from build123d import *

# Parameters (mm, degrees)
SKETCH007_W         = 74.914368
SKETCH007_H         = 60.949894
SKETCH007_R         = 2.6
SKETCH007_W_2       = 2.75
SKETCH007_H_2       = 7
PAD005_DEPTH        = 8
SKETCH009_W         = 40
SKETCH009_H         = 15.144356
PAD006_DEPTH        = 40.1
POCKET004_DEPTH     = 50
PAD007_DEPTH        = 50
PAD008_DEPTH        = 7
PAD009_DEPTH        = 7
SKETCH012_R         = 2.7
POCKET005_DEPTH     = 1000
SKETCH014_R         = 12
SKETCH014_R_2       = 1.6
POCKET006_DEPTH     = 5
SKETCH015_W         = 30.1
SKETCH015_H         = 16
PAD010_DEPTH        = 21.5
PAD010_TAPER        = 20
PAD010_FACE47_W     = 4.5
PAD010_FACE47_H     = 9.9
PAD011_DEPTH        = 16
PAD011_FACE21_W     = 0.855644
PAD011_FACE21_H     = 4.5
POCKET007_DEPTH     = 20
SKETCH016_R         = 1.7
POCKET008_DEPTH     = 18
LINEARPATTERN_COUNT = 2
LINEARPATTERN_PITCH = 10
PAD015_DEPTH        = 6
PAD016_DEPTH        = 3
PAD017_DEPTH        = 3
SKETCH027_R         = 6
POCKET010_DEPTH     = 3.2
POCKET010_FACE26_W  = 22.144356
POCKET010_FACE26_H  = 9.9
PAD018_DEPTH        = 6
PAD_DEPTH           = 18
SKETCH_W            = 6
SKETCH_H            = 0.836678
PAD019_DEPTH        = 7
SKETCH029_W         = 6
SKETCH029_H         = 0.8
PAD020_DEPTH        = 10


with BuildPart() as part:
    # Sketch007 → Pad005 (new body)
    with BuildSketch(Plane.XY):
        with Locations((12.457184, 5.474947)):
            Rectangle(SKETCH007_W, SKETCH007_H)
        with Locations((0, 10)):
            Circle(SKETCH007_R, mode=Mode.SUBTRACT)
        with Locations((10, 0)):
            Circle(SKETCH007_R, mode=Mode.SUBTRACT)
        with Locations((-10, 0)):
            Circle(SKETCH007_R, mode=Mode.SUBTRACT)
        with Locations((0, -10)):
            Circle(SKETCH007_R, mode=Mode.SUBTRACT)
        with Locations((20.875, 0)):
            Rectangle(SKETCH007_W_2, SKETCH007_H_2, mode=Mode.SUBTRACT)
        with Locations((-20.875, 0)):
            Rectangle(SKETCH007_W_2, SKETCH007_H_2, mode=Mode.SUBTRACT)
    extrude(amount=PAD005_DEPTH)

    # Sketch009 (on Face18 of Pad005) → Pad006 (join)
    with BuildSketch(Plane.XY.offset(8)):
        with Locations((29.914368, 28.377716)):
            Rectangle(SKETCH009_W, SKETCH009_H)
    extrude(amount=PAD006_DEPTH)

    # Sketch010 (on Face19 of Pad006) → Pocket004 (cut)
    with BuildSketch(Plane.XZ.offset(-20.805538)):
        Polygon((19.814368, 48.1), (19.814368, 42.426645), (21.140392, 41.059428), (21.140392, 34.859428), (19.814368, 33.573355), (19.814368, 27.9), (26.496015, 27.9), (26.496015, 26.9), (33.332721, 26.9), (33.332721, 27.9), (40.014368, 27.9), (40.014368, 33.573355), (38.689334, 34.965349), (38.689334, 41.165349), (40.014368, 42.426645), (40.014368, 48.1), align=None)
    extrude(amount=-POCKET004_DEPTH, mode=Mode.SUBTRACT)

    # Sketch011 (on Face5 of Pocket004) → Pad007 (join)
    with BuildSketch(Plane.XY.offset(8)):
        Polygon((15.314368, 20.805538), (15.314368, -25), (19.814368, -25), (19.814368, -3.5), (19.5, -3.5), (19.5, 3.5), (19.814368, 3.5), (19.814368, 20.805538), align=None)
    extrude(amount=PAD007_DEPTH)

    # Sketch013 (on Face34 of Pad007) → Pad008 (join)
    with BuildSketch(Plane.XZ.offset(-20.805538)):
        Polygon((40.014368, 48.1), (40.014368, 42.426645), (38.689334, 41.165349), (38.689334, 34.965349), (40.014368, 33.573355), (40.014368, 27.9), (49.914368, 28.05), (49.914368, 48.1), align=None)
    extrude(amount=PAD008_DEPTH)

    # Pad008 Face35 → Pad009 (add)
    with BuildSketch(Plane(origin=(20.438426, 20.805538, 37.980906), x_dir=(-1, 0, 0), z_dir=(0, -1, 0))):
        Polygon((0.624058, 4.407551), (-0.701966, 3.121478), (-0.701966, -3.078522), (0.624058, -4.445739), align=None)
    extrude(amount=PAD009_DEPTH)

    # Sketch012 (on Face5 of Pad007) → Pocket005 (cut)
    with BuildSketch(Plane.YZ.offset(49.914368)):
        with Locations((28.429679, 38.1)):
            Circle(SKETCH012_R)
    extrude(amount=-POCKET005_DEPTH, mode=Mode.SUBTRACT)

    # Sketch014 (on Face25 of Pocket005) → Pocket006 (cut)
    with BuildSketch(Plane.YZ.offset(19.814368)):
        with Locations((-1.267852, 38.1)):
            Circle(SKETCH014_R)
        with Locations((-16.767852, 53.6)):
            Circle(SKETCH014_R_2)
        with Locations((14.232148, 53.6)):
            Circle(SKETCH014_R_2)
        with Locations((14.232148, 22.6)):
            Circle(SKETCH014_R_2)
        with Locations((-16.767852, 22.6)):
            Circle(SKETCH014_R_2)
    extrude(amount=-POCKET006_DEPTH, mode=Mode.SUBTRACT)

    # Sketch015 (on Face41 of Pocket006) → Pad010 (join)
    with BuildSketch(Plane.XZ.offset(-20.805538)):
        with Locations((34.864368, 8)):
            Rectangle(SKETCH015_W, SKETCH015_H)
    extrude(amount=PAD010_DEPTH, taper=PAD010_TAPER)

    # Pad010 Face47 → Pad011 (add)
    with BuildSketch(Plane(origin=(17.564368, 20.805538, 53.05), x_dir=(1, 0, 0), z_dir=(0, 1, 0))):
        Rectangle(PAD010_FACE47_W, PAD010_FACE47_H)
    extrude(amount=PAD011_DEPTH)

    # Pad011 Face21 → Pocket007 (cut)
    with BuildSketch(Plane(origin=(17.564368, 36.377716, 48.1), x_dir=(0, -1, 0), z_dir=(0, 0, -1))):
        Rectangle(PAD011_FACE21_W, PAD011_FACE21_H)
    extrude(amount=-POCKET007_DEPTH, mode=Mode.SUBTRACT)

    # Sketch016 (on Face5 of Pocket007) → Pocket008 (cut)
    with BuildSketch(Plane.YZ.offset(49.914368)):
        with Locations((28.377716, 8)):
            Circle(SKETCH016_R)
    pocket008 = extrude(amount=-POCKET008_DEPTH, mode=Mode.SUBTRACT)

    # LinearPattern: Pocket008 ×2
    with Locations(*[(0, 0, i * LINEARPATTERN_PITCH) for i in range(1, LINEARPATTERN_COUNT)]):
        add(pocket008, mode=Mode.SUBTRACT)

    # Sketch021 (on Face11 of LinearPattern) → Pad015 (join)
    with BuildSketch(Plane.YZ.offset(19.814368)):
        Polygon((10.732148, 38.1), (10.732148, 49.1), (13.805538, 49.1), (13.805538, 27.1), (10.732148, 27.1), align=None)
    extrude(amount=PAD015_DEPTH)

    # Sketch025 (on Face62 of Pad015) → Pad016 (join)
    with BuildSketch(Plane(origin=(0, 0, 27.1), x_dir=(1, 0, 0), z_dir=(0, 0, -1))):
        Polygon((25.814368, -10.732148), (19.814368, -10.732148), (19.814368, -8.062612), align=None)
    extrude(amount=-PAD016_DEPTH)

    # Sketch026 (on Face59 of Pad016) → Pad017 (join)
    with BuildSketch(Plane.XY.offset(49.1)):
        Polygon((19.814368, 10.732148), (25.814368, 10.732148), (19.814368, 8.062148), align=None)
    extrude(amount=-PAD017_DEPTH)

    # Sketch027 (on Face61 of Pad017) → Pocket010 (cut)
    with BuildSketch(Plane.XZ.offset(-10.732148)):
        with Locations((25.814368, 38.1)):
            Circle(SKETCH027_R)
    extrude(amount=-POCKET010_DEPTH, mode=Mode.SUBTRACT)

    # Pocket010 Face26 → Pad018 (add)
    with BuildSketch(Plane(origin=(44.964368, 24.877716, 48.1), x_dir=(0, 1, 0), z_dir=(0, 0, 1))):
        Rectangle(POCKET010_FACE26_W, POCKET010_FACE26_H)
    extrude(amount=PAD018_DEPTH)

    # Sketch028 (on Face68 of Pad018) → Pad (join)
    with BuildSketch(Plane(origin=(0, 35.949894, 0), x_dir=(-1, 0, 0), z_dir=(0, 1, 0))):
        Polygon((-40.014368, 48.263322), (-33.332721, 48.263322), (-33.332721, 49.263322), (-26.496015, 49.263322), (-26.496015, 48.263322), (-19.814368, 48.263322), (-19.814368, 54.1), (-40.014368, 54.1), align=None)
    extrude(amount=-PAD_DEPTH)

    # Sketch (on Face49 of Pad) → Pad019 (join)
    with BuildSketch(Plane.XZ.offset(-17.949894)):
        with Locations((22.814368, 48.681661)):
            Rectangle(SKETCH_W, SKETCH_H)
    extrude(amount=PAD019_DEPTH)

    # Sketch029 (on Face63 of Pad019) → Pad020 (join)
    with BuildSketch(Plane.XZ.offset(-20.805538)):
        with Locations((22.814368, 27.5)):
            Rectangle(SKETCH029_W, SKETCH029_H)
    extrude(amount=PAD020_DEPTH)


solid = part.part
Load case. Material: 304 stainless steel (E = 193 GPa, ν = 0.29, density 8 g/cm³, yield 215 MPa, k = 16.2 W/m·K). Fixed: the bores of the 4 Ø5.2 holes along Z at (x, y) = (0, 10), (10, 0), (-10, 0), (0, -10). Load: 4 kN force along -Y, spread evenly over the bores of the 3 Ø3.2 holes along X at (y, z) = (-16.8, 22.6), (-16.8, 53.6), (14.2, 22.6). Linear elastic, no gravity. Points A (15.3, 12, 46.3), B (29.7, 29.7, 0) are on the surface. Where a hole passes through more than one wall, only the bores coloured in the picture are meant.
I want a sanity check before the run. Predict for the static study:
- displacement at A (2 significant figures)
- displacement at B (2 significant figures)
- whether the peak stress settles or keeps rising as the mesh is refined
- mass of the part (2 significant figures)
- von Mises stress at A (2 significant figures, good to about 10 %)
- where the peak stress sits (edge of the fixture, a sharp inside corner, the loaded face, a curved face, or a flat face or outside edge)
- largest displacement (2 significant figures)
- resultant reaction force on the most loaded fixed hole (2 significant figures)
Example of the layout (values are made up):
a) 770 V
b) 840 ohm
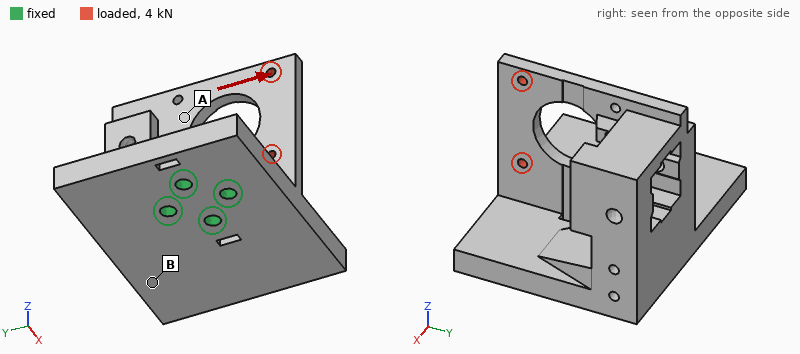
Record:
a) 66 µm
b) 42 µm
c) keeps rising
d) 550 g
e) 31 MPa
f) edge of the fixture
g) 99 µm
h) 3.6 kN
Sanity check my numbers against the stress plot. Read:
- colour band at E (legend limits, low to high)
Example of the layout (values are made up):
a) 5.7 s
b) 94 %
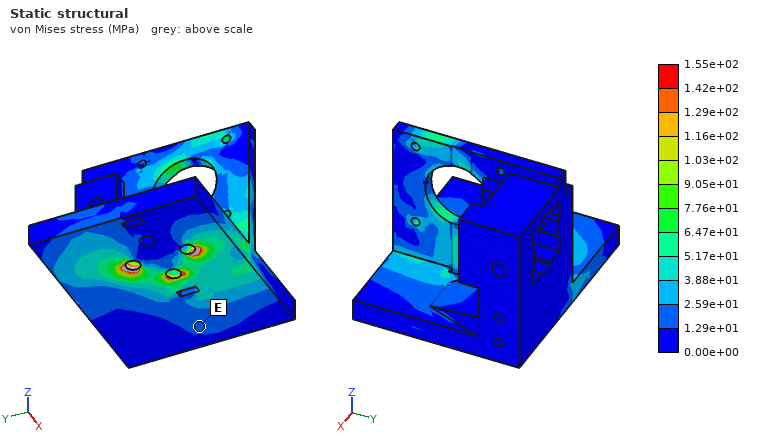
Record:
a) 1.29e+01 to 2.59e+01 MPa
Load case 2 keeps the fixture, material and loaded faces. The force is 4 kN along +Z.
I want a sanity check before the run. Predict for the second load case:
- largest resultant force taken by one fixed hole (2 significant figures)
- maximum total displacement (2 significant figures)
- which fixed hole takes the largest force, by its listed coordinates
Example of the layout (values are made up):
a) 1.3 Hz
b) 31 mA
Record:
a) 3.6 kN
b) 32 µm
c) (10, 0)
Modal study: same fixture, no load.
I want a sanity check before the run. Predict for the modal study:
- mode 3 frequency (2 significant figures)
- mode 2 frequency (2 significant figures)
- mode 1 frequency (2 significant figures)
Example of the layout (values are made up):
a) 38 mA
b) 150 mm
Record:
a) 2900 Hz
b) 2500 Hz
c) 1300 Hz
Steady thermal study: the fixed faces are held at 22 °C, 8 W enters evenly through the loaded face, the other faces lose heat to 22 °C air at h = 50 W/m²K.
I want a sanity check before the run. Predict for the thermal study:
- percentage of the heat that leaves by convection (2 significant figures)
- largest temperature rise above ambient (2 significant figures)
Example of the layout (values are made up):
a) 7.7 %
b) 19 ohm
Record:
a) 75 %
b) 46 K
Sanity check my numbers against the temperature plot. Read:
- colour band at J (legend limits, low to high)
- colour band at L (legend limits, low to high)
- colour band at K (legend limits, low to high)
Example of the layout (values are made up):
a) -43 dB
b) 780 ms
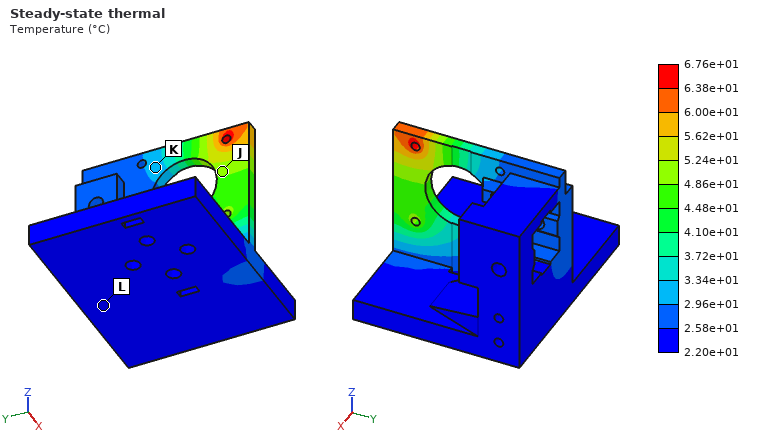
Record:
a) 4.86e+01 to 5.24e+01 °C
b) 2.20e+01 to 2.58e+01 °C
c) 2.96e+01 to 3.34e+01 °C
